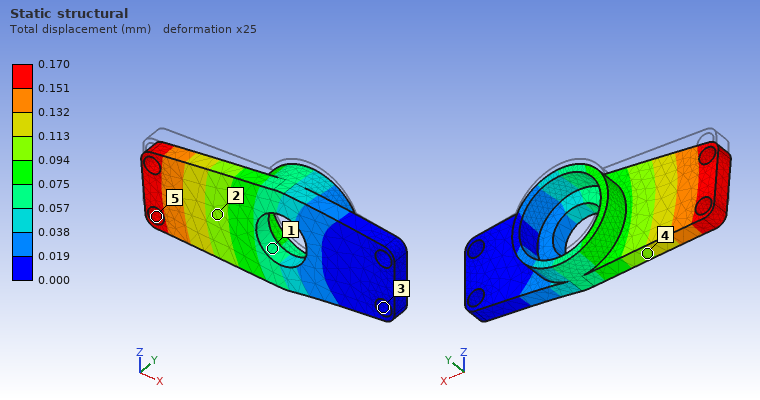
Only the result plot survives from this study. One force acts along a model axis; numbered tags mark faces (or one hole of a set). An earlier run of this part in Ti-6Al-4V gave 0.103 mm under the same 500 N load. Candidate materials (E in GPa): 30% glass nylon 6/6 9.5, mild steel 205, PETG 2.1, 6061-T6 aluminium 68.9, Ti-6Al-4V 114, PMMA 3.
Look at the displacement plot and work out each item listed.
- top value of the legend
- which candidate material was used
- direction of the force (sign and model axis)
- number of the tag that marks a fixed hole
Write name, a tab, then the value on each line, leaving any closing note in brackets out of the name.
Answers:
top value of the legend	0.170 mm
which candidate material was used	6061-T6 aluminium
direction of the force	-Z
number of the tag that marks a fixed hole	3
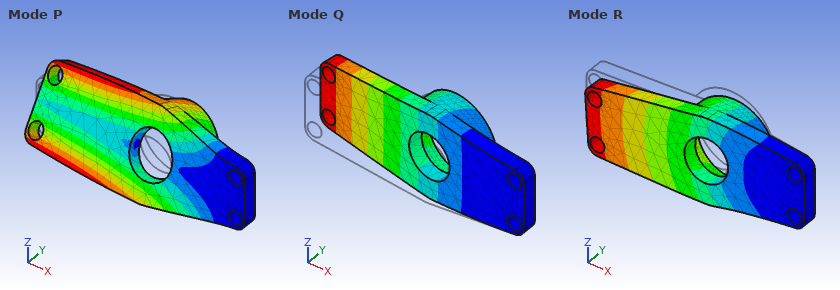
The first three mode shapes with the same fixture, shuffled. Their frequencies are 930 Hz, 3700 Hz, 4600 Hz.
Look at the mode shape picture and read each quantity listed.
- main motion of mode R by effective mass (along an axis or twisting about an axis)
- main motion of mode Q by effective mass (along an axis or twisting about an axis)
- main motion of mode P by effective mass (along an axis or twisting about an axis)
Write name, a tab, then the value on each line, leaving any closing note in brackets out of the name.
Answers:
main motion of mode R by effective mass	along Z
main motion of mode Q by effective mass	along Y
main motion of mode P by effective mass	twisting about X
